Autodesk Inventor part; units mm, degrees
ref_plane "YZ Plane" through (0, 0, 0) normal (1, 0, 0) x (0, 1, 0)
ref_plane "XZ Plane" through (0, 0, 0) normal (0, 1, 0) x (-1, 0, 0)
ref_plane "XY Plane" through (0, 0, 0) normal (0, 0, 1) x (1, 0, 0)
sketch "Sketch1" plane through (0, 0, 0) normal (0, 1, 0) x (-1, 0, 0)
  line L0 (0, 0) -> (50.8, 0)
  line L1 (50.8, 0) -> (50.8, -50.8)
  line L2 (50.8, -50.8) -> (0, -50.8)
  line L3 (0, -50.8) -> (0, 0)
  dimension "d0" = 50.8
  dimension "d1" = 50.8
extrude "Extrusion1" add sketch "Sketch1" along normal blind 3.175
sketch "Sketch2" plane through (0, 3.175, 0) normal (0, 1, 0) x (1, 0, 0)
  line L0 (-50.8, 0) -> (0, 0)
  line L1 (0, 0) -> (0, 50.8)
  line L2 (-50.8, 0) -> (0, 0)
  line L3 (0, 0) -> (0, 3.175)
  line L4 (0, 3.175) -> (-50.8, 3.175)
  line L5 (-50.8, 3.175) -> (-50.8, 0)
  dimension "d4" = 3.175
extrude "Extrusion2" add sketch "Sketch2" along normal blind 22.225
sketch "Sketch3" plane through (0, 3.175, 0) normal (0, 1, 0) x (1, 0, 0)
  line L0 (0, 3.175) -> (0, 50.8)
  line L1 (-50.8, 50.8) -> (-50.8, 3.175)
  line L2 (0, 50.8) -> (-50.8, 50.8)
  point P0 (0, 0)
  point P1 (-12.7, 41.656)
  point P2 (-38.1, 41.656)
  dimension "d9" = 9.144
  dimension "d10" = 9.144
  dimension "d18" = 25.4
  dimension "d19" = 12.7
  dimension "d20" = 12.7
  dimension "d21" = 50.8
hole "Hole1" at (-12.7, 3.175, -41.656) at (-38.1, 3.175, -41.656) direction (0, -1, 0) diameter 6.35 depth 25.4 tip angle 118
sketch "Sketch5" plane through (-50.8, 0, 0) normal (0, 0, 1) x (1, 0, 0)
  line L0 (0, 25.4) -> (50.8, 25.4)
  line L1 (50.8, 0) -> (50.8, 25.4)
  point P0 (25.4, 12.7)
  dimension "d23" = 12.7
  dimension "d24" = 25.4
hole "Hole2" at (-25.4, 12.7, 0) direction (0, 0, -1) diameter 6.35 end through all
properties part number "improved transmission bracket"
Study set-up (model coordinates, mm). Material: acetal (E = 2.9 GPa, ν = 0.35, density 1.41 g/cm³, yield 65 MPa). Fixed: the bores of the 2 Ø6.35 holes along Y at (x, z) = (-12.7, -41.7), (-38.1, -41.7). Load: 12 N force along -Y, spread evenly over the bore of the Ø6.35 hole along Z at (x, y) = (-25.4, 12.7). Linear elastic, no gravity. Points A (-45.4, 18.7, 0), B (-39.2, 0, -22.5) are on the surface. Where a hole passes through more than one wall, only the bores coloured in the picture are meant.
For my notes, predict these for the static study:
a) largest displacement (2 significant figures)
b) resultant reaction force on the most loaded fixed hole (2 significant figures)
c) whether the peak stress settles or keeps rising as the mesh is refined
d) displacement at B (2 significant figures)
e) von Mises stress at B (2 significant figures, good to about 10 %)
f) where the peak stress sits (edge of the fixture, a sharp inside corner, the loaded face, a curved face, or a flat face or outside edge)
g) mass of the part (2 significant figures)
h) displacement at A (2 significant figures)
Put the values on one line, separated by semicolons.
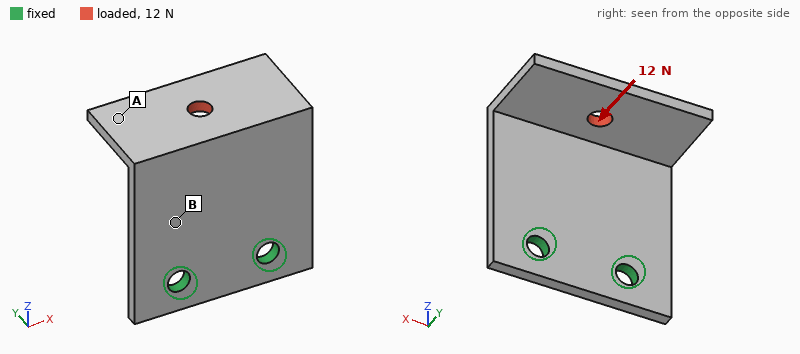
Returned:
0.78 mm; 6.0 N; keeps rising; 0.16 mm; 2.6 MPa; edge of the fixture; 16 g; 0.70 mm
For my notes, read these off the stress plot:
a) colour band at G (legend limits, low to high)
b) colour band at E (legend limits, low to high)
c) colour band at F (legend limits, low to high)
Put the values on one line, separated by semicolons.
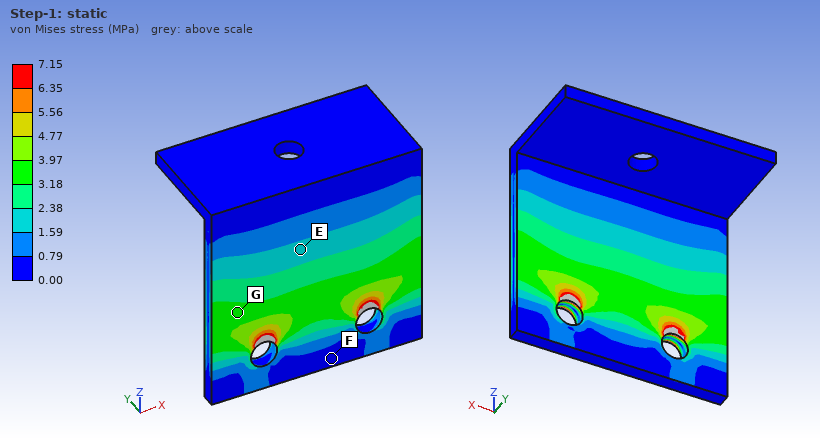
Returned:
3.18 to 3.97 MPa; 1.59 to 2.38 MPa; 0.00 to 0.79 MPa
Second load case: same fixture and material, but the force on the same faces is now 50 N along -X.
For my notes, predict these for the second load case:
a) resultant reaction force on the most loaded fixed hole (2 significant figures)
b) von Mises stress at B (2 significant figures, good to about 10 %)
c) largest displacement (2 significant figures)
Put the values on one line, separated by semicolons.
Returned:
72 N; 3.4 MPa; 0.79 mm
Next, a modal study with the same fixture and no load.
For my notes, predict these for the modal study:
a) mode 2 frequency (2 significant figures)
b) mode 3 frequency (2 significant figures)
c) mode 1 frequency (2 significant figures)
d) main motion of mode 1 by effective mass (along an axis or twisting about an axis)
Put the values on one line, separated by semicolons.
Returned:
480 Hz; 870 Hz; 250 Hz; along Y
